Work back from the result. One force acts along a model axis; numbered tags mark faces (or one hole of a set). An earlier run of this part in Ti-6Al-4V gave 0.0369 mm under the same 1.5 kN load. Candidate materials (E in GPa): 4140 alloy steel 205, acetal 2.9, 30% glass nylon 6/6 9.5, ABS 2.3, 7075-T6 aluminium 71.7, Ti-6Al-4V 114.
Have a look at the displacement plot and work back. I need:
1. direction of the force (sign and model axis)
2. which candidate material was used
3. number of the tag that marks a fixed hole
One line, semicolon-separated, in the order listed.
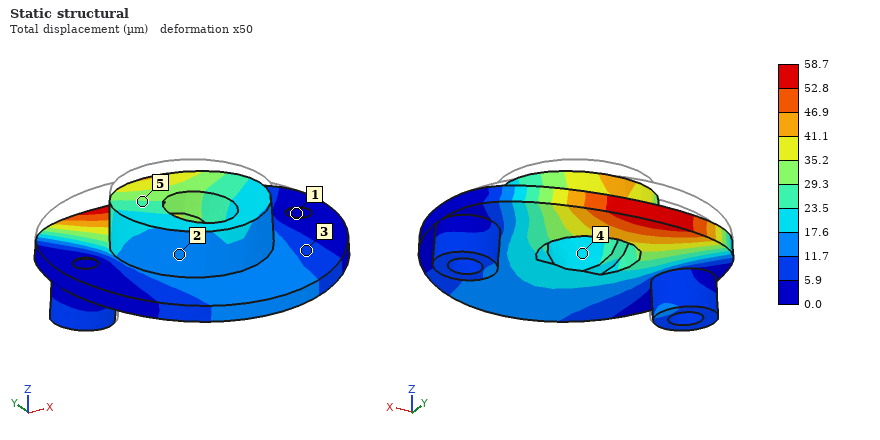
-Z; 7075-T6 aluminium; 1
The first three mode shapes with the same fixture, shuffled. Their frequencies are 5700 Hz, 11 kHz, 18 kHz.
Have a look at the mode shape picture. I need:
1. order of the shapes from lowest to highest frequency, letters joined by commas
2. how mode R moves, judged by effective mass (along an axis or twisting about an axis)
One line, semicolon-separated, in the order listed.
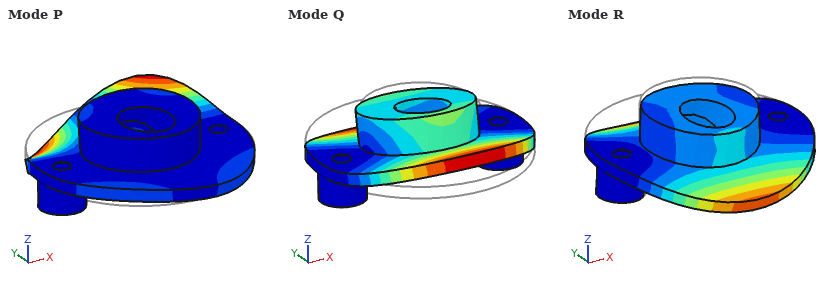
Q, R, P; along Z
